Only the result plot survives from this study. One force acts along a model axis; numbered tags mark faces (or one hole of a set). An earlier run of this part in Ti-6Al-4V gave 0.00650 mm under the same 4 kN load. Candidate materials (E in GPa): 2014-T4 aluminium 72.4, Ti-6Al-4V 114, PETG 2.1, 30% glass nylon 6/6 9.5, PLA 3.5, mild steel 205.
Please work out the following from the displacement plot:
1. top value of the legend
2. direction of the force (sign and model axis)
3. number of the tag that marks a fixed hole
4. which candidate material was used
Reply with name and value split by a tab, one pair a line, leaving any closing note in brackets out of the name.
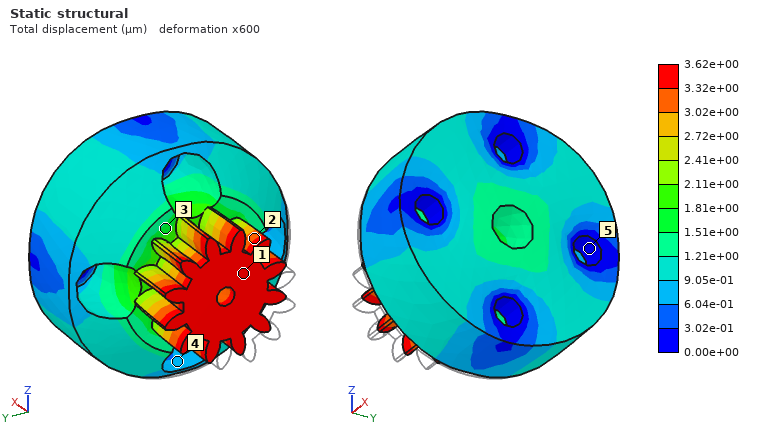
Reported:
top value of the legend	3.62e+00 µm
direction of the force	+X
number of the tag that marks a fixed hole	5
which candidate material was used	mild steel
